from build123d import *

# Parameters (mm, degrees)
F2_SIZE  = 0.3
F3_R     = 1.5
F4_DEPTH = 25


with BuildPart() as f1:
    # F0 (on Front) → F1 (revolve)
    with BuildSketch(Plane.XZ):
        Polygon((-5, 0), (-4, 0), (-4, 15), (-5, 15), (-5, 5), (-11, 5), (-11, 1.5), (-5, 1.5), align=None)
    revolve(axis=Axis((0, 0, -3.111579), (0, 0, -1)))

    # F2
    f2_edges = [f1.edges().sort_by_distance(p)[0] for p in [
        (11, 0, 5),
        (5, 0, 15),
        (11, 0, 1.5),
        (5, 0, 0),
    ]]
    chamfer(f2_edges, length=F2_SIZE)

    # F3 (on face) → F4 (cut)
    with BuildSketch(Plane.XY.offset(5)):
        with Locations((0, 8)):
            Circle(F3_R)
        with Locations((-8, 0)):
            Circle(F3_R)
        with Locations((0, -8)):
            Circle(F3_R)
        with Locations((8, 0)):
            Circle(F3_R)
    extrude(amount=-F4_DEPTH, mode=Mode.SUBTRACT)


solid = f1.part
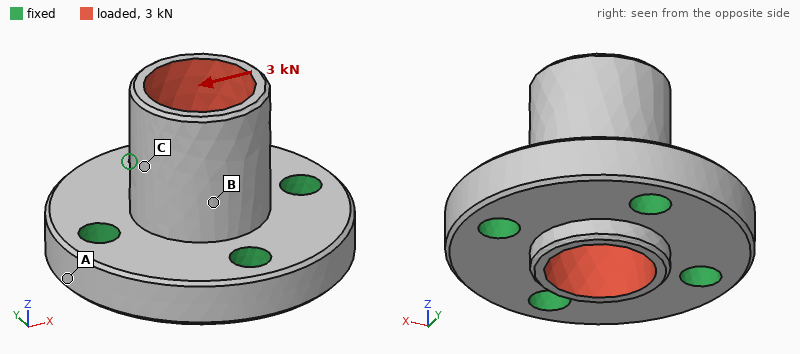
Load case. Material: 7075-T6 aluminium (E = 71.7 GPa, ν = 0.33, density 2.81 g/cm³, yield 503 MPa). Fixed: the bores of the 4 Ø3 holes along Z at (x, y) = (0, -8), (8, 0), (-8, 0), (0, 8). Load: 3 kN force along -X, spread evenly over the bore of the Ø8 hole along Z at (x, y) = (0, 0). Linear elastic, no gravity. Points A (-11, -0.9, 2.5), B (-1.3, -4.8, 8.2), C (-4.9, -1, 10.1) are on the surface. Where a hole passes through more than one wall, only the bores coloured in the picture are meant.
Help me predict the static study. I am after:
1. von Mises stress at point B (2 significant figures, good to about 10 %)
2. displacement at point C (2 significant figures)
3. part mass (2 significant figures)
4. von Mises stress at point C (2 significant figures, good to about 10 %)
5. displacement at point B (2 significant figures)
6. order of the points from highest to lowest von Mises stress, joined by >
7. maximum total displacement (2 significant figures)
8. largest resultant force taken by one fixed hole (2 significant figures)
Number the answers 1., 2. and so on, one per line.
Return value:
1. 140 MPa
2. 38 µm
3. 3.9 g
4. 54 MPa
5. 22 µm
6. B > C > A
7. 57 µm
8. 1.2 kN
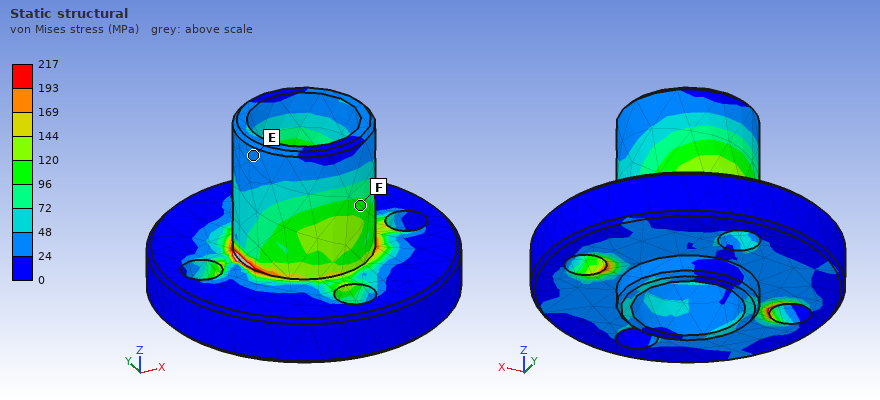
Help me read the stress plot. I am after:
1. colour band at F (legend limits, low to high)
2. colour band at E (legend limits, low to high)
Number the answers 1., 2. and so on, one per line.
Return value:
1. 96 to 120 MPa
2. 24 to 48 MPa
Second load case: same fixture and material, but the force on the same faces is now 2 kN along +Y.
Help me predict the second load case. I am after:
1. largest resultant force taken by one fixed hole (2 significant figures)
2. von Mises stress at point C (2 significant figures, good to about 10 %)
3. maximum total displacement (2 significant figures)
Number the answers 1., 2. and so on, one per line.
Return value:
1. 830 N
2. 73 MPa
3. 38 µm
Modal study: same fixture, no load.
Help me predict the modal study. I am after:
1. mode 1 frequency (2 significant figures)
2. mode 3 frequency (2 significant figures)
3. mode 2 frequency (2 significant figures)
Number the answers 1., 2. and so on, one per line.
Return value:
1. 39 kHz
2. 40 kHz
3. 39 kHz
